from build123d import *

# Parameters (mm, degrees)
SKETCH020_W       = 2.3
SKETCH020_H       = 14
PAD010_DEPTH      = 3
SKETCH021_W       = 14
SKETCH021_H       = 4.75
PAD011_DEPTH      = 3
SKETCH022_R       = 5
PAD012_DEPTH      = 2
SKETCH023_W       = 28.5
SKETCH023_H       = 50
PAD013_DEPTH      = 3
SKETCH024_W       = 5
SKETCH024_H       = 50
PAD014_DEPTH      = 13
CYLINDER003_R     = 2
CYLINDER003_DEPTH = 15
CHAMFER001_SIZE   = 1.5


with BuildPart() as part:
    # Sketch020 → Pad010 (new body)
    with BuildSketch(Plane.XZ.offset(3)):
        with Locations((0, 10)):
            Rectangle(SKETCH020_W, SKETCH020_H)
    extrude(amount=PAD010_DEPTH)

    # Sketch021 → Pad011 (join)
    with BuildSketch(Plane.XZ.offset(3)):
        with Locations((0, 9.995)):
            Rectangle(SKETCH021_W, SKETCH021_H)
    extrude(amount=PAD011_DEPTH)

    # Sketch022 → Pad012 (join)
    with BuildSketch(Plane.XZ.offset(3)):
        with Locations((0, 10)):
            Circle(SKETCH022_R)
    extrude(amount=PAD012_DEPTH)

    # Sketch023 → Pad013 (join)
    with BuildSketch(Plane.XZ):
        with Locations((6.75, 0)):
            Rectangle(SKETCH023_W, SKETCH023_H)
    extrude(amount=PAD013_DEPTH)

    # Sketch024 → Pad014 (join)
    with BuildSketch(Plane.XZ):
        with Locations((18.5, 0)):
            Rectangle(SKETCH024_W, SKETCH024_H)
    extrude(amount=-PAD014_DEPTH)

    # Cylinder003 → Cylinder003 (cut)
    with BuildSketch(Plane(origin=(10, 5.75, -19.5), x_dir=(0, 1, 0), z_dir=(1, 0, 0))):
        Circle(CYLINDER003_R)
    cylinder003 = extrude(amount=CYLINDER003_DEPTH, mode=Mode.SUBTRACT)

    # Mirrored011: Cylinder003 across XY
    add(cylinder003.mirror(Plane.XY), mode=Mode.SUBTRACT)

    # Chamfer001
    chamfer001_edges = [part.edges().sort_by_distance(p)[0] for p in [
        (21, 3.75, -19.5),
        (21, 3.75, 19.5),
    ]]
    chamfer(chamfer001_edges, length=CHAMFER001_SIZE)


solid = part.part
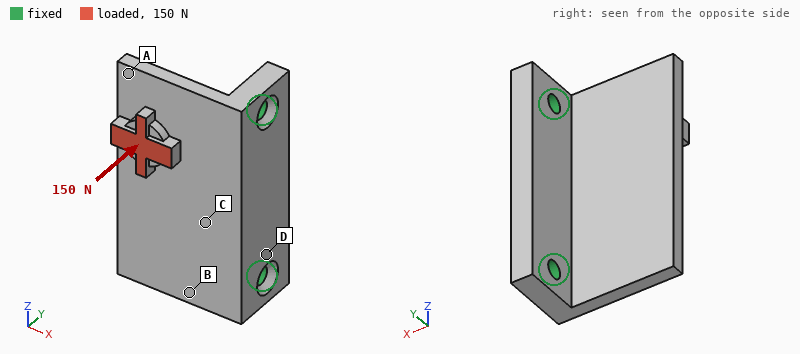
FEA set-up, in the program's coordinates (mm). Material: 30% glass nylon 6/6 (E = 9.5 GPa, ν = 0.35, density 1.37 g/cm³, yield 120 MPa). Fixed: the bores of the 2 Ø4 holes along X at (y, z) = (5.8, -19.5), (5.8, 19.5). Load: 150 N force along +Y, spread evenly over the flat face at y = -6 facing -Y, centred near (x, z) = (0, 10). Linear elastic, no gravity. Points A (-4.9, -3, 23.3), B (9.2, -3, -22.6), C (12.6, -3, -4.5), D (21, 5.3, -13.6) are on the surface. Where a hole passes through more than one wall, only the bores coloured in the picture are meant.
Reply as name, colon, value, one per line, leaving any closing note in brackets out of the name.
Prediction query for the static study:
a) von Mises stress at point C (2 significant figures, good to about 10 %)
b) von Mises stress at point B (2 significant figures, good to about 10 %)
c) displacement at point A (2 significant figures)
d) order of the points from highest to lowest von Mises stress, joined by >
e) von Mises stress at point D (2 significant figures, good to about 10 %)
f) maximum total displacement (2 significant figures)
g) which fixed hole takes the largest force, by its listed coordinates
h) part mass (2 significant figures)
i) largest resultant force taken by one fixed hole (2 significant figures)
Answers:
von Mises stress at point C: 21 MPa
von Mises stress at point B: 15 MPa
displacement at point A: 0.61 mm
order of the points from highest to lowest von Mises stress, joined by >: C > B > D > A
von Mises stress at point D: 8.9 MPa
maximum total displacement: 0.70 mm
which fixed hole takes the largest force, by its listed coordinates: (5.8, 19.5)
part mass: 11 g
largest resultant force taken by one fixed hole: 110 N
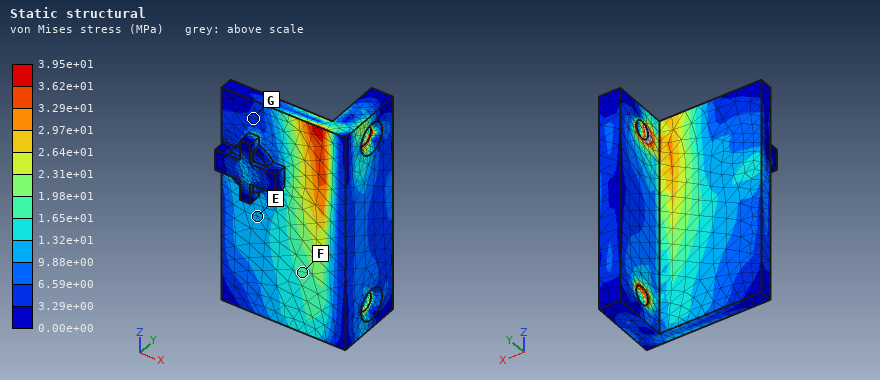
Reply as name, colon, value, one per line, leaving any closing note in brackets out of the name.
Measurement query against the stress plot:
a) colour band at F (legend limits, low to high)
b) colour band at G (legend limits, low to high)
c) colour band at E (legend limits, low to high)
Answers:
colour band at F: 1.65e+01 to 1.98e+01 MPa
colour band at G: 3.29e+00 to 6.59e+00 MPa
colour band at E: 9.88e+00 to 1.32e+01 MPa
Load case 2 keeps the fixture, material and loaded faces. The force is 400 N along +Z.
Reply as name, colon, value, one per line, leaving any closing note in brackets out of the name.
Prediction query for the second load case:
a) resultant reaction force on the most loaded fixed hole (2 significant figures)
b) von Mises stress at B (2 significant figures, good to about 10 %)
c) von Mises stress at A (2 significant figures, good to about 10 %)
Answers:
resultant reaction force on the most loaded fixed hole: 300 N
von Mises stress at B: 4.6 MPa
von Mises stress at A: 4.5 MPa
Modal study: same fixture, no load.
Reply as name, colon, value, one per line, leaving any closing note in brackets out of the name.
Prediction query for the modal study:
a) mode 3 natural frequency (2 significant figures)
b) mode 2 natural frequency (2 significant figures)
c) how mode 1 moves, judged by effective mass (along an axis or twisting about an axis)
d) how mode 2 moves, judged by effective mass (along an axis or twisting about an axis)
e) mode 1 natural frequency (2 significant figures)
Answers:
mode 3 natural frequency: 5800 Hz
mode 2 natural frequency: 2900 Hz
how mode 1 moves, judged by effective mass: along Y
how mode 2 moves, judged by effective mass: twisting about X
mode 1 natural frequency: 1600 Hz
